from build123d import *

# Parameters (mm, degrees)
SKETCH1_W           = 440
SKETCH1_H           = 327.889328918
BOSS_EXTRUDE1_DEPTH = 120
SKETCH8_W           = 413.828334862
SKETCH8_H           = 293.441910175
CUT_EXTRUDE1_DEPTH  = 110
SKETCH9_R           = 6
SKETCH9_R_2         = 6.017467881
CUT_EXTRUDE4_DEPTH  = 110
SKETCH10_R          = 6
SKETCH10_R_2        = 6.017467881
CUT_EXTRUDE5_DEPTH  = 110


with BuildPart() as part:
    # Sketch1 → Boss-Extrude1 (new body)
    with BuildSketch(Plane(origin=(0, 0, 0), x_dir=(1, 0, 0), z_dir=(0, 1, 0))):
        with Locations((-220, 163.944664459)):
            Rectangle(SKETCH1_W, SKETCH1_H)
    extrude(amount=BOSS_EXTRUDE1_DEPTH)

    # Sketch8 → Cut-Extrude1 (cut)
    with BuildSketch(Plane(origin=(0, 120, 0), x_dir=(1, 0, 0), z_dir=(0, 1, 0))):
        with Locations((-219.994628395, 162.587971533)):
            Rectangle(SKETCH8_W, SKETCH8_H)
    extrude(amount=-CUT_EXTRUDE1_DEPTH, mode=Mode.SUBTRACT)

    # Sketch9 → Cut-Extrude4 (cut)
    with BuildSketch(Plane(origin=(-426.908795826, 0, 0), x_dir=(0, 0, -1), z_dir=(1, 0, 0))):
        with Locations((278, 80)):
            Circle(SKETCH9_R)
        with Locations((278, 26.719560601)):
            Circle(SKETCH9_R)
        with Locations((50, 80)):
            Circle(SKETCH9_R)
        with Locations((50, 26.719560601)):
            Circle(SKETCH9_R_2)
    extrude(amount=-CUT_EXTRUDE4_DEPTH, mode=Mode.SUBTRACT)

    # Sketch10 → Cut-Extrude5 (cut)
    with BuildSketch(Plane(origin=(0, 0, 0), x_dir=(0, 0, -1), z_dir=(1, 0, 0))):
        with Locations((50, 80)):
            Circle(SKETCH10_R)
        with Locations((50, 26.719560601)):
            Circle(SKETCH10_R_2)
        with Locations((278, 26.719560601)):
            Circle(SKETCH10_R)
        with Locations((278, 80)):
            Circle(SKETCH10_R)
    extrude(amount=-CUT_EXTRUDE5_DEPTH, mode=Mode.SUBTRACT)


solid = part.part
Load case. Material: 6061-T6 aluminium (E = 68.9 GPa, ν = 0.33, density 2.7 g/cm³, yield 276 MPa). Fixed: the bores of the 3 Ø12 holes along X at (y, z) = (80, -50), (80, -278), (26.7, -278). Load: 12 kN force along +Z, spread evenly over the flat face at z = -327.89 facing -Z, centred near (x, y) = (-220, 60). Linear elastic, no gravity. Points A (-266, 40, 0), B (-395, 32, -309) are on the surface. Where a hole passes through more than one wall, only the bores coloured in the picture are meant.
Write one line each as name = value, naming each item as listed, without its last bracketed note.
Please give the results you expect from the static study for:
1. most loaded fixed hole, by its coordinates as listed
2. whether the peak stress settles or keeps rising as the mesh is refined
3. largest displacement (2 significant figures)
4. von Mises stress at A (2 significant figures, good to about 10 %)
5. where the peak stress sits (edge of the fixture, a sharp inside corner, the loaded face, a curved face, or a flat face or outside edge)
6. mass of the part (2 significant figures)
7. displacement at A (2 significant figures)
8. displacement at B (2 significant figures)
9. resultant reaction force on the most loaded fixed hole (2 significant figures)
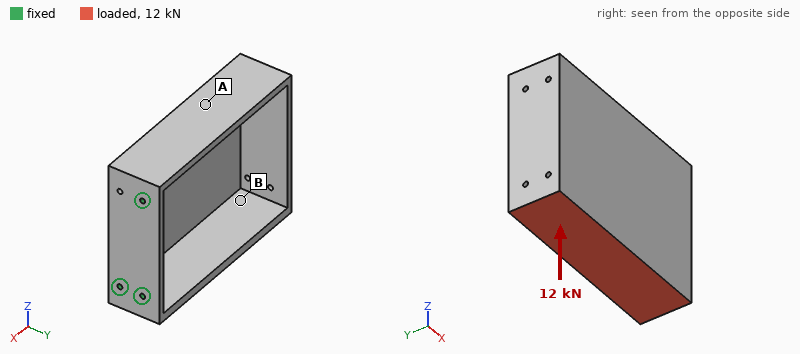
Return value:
most loaded fixed hole, by its coordinates as listed = (80, -50)
whether the peak stress settles or keeps rising as the mesh is refined = keeps rising
largest displacement = 4.0 mm
von Mises stress at A = 20 MPa
where the peak stress sits = edge of the fixture
mass of the part = 11 kg
displacement at A = 2.2 mm
displacement at B = 1.3 mm
resultant reaction force on the most loaded fixed hole = 9.9 kN
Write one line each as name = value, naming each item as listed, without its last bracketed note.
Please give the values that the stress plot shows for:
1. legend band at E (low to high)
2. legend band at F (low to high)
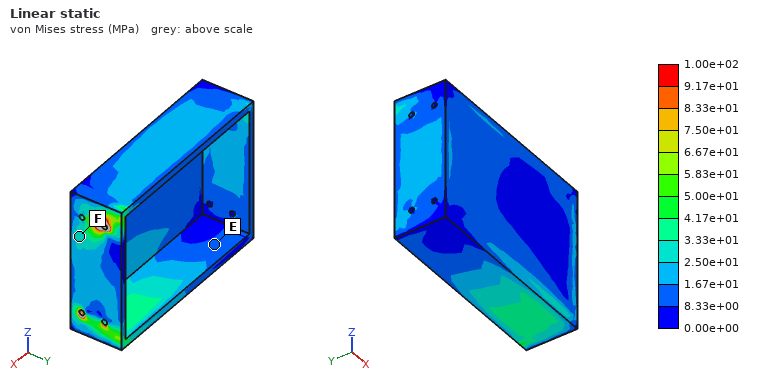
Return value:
legend band at E = 8.33e+00 to 1.67e+01 MPa
legend band at F = 2.50e+01 to 3.33e+01 MPa
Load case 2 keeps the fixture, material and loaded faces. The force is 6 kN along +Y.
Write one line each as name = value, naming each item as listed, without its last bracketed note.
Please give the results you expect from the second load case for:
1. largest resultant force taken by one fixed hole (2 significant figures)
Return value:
largest resultant force taken by one fixed hole = 17 kN
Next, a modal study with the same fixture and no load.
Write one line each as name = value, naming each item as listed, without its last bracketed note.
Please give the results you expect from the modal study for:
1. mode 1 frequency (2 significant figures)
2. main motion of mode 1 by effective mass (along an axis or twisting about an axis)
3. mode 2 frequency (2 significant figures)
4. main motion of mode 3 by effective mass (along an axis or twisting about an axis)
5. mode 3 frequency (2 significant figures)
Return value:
mode 1 frequency = 90 Hz
main motion of mode 1 by effective mass = along Y
mode 2 frequency = 170 Hz
main motion of mode 3 by effective mass = along Z
mode 3 frequency = 400 Hz
